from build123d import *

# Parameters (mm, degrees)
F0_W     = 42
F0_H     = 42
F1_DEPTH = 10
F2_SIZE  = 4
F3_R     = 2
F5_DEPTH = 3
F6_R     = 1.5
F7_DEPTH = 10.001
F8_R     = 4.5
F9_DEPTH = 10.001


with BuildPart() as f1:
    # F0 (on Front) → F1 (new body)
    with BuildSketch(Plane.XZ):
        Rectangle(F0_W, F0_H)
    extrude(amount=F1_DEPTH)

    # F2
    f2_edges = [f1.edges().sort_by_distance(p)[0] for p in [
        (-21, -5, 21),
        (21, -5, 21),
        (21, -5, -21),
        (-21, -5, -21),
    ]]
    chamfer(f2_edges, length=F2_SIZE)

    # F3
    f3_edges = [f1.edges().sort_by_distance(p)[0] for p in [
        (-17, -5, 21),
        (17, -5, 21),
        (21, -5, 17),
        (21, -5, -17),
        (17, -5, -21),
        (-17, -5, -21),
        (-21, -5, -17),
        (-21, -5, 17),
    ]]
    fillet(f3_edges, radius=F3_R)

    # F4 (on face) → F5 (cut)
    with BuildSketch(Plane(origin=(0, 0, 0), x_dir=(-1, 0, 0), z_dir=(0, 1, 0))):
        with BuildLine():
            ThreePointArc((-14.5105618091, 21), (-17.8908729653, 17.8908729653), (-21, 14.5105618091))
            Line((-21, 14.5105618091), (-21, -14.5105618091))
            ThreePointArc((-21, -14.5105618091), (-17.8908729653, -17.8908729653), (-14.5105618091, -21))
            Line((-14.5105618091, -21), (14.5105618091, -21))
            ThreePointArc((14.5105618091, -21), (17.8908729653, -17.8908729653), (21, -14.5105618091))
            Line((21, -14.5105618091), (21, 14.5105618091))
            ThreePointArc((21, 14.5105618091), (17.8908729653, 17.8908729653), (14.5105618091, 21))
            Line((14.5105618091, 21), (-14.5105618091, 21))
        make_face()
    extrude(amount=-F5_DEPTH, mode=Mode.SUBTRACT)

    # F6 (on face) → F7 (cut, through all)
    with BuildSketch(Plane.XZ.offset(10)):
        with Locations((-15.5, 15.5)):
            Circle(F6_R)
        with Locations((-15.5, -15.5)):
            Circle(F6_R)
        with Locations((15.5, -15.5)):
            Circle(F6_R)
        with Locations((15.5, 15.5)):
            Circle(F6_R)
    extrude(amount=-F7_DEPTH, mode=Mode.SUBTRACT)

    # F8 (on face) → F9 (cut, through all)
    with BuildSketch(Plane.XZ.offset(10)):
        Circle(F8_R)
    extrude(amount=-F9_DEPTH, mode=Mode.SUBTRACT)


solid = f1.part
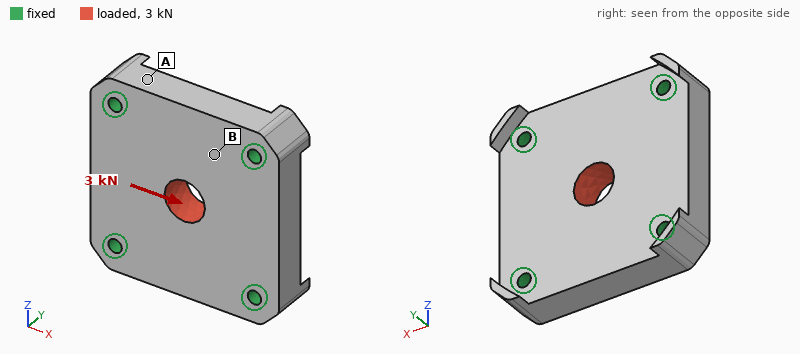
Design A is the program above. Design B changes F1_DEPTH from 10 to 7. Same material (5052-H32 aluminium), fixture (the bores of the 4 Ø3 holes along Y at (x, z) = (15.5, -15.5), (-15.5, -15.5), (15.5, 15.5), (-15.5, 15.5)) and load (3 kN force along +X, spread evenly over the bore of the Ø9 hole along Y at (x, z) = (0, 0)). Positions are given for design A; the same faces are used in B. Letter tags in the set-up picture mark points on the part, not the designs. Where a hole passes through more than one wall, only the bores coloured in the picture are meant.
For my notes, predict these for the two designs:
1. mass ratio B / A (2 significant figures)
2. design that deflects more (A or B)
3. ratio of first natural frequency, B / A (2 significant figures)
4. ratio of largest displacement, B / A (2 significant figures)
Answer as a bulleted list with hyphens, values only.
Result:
- 0.58
- B
- 0.68
- 1.7
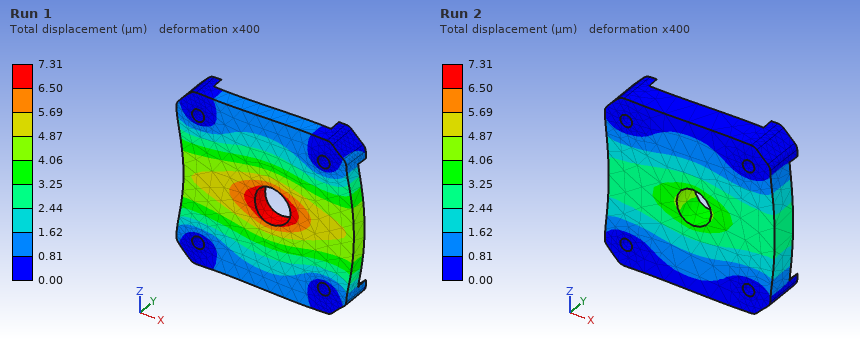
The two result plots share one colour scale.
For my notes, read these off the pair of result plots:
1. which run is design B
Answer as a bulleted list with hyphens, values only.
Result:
- Run 1
